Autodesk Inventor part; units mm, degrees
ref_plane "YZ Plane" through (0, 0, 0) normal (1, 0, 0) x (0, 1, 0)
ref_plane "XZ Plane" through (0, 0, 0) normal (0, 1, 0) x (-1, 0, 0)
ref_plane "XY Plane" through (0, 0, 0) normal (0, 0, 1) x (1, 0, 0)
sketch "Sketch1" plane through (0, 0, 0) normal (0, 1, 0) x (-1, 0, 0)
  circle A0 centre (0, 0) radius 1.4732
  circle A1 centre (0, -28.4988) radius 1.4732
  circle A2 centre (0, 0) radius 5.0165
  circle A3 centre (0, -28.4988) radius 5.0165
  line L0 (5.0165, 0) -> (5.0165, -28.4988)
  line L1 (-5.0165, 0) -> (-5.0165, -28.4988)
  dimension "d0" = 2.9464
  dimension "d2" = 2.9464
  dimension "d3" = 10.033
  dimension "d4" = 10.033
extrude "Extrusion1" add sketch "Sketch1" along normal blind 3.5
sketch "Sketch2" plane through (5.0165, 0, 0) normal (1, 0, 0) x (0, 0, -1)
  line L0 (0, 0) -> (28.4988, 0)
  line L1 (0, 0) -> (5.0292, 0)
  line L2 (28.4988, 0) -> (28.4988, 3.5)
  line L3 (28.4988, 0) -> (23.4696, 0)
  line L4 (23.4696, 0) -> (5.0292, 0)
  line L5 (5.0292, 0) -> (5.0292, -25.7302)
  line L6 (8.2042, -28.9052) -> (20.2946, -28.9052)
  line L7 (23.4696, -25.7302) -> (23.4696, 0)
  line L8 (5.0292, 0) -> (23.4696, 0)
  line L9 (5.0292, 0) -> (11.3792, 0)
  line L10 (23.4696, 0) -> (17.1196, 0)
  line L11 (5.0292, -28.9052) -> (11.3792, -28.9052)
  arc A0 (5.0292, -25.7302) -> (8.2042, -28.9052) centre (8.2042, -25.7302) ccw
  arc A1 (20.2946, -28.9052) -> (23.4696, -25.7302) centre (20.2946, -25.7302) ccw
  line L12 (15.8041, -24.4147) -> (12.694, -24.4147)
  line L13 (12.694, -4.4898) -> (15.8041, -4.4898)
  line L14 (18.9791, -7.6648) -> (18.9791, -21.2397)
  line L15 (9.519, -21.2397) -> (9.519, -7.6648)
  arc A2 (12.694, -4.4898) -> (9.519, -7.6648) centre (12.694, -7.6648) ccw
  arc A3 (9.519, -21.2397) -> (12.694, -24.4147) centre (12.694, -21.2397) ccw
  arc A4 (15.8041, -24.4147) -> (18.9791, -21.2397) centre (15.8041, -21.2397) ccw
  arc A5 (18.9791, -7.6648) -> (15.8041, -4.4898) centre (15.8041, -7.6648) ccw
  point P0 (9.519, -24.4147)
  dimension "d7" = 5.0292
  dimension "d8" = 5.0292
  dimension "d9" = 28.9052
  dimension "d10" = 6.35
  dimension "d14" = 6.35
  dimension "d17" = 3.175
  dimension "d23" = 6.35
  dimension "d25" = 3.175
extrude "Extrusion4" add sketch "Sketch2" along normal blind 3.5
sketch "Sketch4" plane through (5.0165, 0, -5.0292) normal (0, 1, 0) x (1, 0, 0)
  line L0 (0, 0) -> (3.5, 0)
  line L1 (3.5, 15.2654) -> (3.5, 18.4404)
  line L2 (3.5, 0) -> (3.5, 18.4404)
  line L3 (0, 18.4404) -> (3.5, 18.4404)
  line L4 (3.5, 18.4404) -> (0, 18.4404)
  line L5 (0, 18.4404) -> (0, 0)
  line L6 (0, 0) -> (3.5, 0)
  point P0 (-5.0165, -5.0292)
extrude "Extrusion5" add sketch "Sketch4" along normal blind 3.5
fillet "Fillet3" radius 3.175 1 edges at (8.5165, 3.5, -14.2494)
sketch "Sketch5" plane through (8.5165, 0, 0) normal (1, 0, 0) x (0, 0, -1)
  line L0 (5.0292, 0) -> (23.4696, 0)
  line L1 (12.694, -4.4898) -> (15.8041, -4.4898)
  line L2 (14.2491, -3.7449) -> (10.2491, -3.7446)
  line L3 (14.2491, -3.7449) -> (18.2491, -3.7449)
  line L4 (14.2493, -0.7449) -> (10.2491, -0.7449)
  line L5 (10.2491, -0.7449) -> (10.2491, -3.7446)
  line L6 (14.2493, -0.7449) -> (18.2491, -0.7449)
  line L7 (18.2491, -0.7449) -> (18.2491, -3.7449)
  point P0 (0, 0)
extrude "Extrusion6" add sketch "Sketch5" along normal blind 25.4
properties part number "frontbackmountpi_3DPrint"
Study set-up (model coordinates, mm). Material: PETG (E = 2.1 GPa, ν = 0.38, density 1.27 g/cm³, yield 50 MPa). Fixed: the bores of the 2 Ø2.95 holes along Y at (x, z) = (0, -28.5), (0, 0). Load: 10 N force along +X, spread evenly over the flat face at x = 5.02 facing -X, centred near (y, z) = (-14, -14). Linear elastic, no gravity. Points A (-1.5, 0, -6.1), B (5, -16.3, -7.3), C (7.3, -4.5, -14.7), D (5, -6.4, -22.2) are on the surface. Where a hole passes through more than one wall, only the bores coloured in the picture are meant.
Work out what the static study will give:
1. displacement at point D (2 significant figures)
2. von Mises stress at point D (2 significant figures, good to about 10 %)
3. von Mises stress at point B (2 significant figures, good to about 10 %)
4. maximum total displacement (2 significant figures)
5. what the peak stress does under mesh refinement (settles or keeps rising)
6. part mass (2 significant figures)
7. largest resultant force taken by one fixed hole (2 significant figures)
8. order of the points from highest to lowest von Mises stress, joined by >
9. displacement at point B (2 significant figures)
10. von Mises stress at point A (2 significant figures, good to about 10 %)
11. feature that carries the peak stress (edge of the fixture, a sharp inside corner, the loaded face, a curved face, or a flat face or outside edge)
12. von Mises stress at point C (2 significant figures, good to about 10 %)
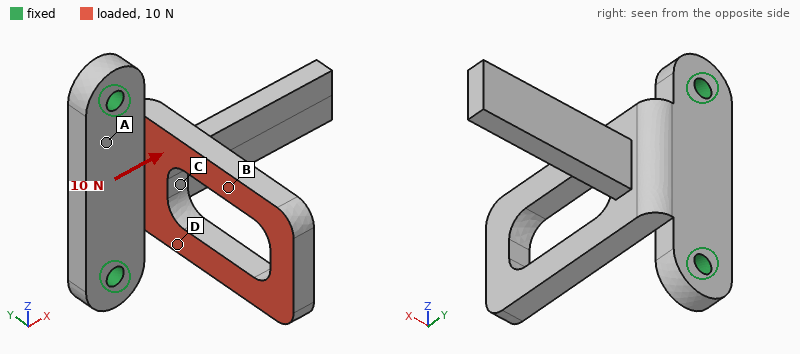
0.12 mm
4.2 MPa
1.8 MPa
0.74 mm
keeps rising
4.1 g
5.3 N
D > A > B > C
0.36 mm
2.6 MPa
a sharp inside corner
0.95 MPa
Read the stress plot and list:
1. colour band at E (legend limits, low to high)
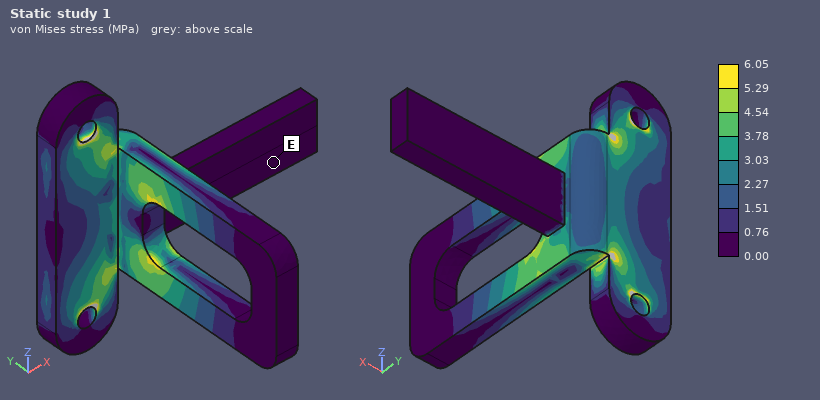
0.00 to 0.76 MPa
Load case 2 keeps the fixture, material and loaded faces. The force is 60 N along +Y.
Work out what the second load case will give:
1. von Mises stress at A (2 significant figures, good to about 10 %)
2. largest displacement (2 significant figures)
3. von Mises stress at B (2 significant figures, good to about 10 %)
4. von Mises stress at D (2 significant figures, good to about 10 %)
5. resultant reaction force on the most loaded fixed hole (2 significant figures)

3.5 MPa
0.36 mm
3.4 MPa
5.2 MPa
30 N
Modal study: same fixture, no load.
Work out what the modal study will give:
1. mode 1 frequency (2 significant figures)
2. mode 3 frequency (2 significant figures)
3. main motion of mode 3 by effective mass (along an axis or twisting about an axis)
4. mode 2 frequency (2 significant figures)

490 Hz
1400 Hz
along Z
860 Hz
